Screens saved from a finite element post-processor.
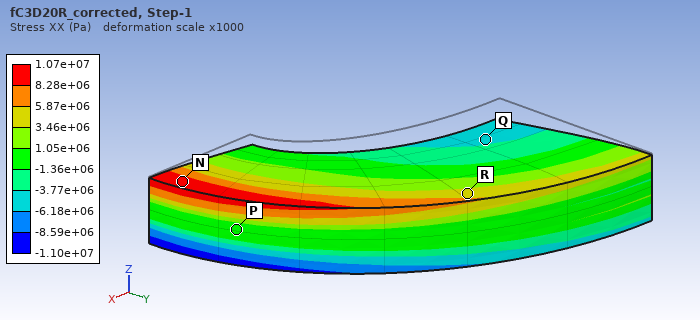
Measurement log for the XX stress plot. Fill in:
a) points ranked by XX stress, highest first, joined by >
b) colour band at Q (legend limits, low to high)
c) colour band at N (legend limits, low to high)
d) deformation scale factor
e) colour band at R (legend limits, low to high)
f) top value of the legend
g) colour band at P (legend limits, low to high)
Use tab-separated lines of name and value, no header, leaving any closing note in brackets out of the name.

points ranked by XX stress, highest first, joined by >	N > R > P > Q
colour band at Q	-6.18e+06 to -3.77e+06 Pa
colour band at N	8.28e+06 to 1.07e+07 Pa
deformation scale factor	1000
colour band at R	3.46e+06 to 5.87e+06 Pa
top value of the legend	1.07e+07 Pa
colour band at P	-1.36e+06 to 1.05e+06 Pa
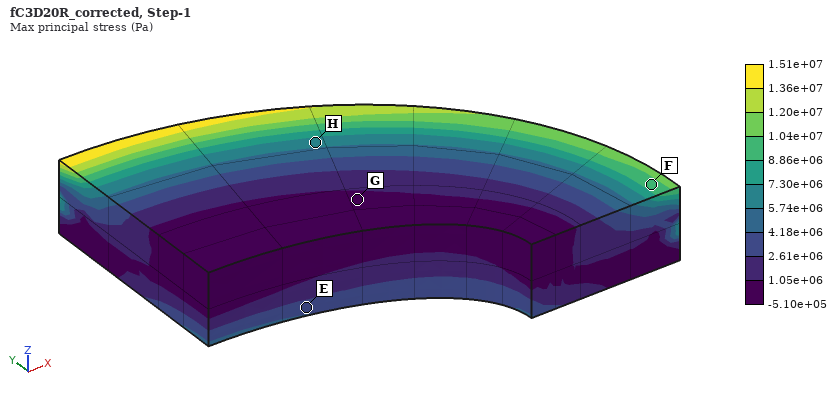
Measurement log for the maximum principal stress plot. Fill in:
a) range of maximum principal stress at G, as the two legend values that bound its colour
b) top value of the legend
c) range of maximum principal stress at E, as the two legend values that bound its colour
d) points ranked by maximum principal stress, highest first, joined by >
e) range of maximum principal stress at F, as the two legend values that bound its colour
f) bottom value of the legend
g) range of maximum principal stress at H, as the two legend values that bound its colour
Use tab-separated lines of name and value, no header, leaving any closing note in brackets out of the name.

range of maximum principal stress at G, as the two legend values that bound its colour	-5.10e+05 to 1.05e+06 Pa
top value of the legend	1.51e+07 Pa
range of maximum principal stress at E, as the two legend values that bound its colour	2.61e+06 to 4.18e+06 Pa
points ranked by maximum principal stress, highest first, joined by >	F > H > E > G
range of maximum principal stress at F, as the two legend values that bound its colour	8.86e+06 to 1.04e+07 Pa
bottom value of the legend	-5.10e+05 Pa
range of maximum principal stress at H, as the two legend values that bound its colour	5.74e+06 to 7.30e+06 Pa
